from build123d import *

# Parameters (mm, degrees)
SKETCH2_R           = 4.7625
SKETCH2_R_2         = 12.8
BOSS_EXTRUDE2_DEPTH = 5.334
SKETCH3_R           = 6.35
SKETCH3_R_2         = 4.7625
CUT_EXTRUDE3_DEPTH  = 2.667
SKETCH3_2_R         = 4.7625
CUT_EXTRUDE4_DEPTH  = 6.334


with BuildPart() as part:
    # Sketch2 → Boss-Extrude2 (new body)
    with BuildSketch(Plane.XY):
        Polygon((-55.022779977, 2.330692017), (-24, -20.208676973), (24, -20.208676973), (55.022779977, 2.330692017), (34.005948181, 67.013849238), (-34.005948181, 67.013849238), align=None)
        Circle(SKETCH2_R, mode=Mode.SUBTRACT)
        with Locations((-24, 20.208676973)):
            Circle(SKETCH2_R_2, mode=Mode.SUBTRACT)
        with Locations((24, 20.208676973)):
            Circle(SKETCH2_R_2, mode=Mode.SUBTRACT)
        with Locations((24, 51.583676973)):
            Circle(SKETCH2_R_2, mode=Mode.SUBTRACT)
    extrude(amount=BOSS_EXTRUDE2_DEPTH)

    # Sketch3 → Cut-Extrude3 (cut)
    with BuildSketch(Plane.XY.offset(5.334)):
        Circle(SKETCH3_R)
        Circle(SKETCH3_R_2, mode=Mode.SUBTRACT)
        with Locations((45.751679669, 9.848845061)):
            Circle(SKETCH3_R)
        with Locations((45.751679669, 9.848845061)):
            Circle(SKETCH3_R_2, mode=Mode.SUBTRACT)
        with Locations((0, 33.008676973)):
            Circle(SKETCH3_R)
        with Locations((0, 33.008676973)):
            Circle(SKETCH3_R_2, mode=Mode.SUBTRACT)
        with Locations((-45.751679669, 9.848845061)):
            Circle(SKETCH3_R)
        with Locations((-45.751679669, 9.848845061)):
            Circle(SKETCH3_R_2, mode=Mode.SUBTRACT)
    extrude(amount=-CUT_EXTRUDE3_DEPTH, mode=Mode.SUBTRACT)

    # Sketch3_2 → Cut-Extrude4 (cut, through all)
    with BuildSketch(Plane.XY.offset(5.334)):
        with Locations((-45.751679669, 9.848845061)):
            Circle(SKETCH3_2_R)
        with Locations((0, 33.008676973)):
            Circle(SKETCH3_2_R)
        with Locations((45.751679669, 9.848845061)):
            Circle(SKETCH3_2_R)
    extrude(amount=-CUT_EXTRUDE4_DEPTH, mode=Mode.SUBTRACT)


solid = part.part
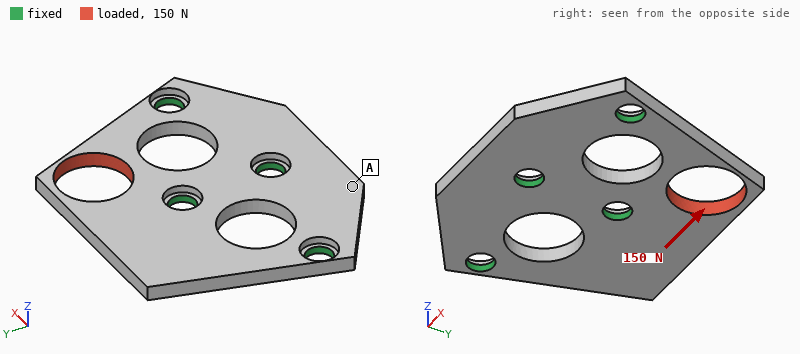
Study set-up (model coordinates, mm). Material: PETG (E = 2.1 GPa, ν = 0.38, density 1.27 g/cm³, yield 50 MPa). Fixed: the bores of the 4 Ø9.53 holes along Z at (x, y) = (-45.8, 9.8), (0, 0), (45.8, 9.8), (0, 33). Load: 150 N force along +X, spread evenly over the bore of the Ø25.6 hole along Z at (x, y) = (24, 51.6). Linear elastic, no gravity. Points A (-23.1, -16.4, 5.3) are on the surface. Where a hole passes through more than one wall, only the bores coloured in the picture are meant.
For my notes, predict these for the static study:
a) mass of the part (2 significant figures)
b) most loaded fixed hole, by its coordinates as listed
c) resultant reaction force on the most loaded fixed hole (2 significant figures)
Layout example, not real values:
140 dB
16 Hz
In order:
38 g
(0, 33)
130 N
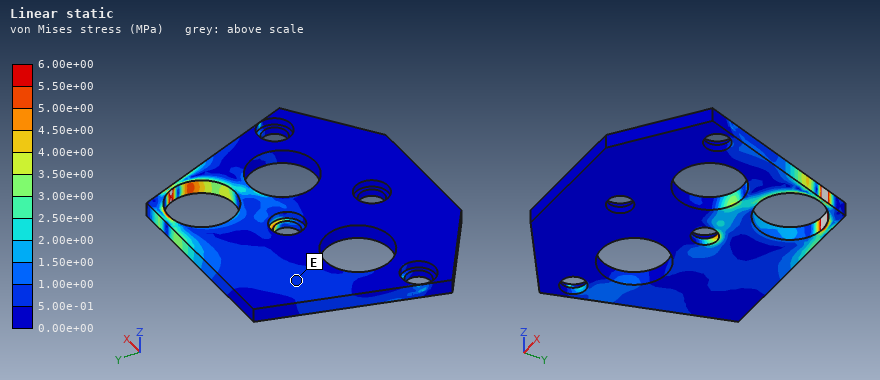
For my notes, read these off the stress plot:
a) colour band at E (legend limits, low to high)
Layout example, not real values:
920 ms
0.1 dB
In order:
5.00e-01 to 1.00e+00 MPa
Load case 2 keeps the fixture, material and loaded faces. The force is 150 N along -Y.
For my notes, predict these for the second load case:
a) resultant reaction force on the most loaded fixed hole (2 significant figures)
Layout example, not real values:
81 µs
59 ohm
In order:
74 N
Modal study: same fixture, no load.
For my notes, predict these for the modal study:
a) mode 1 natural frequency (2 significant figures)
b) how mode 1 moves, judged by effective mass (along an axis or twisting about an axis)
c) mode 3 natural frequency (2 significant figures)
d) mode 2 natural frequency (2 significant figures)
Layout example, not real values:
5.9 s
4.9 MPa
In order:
620 Hz
along Z
1500 Hz
870 Hz
